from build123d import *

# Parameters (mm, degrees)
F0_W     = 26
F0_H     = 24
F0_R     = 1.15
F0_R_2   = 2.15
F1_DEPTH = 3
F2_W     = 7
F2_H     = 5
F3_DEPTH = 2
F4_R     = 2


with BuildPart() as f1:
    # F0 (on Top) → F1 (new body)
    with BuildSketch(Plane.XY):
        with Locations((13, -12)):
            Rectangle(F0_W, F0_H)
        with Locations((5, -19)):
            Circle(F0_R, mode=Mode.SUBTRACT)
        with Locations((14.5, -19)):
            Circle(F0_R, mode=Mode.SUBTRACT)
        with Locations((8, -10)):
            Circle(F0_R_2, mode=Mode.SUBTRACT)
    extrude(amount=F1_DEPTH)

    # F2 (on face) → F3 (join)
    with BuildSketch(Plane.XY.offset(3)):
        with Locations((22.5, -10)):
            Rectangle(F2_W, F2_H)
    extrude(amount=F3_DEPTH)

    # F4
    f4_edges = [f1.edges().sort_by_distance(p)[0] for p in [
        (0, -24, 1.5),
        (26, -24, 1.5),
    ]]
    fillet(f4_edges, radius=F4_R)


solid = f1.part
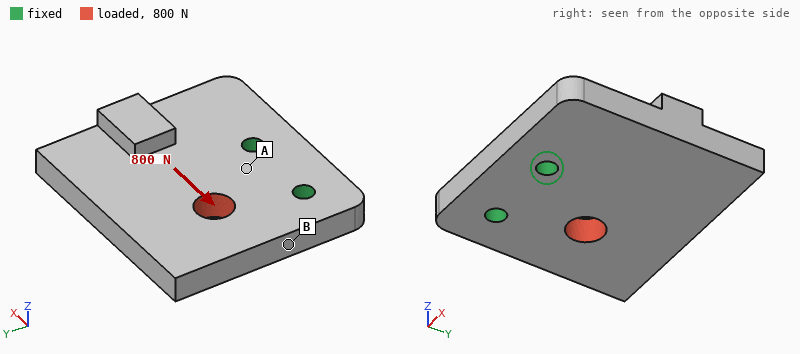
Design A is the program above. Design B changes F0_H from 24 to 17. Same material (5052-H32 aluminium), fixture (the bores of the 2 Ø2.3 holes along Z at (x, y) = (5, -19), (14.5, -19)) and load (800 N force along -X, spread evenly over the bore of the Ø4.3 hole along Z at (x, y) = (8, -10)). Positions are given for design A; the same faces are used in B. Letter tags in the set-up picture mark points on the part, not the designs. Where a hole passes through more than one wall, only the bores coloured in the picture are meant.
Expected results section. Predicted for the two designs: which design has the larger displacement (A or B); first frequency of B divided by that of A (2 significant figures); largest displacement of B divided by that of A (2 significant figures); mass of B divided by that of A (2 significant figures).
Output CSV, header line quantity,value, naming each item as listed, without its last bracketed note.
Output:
quantity,value
which design has the larger displacement,B
first frequency of B divided by that of A,1.3
largest displacement of B divided by that of A,1.1
mass of B divided by that of A,0.71
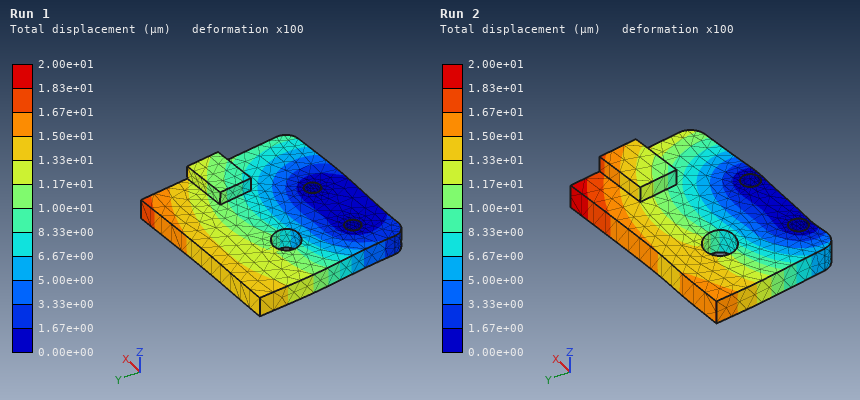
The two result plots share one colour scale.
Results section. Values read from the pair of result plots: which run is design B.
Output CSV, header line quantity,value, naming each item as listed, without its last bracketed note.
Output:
quantity,value
which run is design B,Run 2
